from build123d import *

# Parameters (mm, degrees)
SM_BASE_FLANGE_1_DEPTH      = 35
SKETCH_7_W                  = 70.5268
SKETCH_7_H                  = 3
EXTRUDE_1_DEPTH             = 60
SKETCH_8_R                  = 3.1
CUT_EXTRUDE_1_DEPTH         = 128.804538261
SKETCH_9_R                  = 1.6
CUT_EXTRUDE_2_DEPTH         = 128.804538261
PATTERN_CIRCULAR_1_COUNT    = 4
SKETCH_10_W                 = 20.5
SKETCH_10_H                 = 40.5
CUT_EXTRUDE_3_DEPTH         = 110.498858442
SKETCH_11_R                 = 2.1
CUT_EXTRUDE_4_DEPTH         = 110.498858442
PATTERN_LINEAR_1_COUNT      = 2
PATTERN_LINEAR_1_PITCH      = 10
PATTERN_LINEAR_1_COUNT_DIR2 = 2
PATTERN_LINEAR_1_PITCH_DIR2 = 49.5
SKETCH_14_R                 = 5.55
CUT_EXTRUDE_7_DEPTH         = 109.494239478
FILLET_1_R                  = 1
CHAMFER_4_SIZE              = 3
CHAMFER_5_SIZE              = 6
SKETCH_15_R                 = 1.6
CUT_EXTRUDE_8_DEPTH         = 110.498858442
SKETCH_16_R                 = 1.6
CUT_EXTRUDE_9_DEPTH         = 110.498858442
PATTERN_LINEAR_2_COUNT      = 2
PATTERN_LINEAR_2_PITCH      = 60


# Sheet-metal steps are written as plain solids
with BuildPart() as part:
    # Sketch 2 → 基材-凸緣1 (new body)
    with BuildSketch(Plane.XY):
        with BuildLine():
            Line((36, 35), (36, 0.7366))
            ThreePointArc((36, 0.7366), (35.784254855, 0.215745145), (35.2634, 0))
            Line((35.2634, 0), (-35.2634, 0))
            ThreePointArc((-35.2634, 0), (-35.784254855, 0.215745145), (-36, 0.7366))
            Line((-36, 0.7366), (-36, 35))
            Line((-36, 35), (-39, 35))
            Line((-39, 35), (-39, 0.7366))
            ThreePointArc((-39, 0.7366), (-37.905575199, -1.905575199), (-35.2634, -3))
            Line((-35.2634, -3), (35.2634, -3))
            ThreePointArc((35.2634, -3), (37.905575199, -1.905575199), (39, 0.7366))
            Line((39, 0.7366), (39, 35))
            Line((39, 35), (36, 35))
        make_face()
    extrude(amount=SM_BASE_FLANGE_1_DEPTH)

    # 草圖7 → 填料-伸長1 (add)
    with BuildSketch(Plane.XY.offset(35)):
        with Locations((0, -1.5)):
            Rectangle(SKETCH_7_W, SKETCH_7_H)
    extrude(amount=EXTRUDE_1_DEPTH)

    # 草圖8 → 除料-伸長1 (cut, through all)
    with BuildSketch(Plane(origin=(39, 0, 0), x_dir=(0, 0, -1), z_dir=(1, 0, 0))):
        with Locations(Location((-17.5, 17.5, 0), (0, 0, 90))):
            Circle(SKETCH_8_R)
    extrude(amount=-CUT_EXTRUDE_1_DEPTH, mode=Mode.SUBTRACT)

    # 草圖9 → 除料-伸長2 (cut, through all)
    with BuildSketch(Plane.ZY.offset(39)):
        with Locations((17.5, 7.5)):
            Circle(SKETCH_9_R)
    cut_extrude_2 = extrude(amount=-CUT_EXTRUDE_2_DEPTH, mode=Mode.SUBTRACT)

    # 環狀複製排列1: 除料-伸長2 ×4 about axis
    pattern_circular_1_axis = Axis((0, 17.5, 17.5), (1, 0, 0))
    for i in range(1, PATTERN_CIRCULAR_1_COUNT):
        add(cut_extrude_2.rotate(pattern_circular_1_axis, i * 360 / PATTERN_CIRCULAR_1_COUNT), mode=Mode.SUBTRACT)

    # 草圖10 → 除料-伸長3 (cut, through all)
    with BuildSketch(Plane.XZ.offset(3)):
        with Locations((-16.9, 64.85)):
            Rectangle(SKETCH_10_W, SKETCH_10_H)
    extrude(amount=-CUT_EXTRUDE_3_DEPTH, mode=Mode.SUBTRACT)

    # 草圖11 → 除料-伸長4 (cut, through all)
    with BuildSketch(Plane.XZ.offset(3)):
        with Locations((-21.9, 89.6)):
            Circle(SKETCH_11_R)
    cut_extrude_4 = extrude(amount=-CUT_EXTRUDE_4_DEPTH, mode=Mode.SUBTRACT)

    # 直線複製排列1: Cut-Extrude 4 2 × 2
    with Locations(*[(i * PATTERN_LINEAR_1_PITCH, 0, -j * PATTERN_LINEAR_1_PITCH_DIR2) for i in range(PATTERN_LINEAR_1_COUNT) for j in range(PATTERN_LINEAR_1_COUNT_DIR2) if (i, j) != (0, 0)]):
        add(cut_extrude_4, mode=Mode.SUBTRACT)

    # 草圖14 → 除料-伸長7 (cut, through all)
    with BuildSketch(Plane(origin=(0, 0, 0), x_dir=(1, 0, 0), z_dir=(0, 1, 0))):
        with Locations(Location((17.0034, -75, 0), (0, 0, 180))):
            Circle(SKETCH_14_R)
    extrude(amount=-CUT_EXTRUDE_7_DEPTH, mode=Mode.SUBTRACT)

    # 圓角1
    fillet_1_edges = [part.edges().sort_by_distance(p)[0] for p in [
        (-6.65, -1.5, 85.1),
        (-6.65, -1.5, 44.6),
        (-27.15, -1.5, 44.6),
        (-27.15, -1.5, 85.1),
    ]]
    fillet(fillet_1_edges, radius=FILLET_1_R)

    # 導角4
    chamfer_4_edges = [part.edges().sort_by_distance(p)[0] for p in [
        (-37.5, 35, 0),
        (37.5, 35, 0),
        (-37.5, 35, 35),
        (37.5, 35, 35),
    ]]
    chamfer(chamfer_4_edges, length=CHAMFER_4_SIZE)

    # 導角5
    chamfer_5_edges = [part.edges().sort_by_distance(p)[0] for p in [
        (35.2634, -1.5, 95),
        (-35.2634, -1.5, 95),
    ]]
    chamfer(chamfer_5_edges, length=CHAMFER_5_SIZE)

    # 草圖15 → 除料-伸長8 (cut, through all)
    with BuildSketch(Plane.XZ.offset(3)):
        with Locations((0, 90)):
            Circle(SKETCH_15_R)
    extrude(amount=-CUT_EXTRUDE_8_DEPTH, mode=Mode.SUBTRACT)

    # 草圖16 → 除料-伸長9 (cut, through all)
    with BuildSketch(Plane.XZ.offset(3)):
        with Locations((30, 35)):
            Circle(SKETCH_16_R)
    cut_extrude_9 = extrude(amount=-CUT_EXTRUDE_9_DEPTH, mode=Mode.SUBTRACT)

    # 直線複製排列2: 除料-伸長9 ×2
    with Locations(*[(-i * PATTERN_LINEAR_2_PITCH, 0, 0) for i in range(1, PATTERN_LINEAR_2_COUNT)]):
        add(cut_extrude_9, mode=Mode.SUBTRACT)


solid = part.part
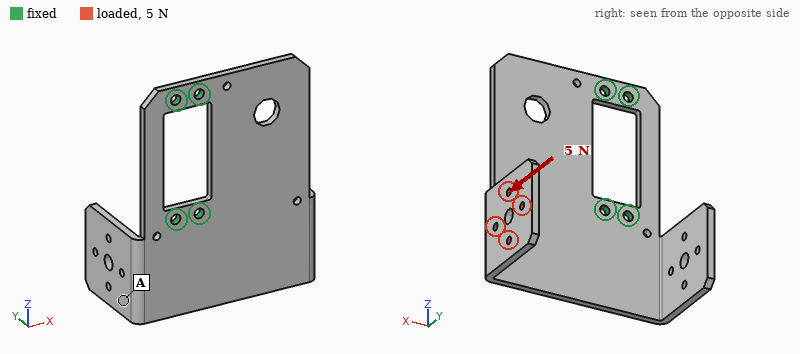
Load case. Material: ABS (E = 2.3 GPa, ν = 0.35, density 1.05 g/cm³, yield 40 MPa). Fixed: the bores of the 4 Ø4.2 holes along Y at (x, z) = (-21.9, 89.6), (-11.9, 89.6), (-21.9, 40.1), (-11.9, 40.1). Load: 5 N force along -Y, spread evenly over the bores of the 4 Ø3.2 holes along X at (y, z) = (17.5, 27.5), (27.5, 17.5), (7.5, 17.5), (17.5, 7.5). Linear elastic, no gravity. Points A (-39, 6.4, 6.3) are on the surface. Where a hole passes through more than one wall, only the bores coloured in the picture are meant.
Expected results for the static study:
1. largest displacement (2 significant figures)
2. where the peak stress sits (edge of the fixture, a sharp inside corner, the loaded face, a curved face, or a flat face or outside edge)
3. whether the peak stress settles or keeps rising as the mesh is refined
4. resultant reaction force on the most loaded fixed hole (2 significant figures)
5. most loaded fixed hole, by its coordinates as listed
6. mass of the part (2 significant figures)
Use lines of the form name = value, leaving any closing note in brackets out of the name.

largest displacement = 1.5 mm
where the peak stress sits = edge of the fixture
whether the peak stress settles or keeps rising as the mesh is refined = keeps rising
resultant reaction force on the most loaded fixed hole = 14 N
most loaded fixed hole, by its coordinates as listed = (-11.9, 40.1)
mass of the part = 26 g
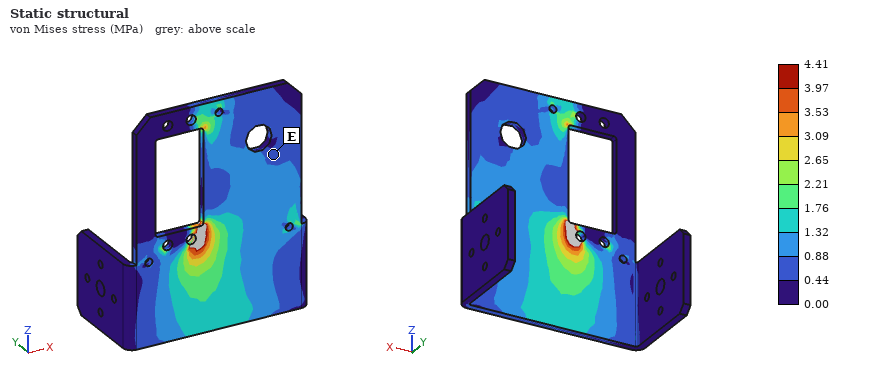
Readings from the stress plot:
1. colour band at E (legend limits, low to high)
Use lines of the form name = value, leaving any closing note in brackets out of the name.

colour band at E = 0.44 to 0.88 MPa
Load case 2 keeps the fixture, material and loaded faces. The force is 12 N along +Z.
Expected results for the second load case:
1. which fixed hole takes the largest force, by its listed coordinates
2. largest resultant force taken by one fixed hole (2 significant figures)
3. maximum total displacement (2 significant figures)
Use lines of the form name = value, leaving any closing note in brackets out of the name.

which fixed hole takes the largest force, by its listed coordinates = (-11.9, 40.1)
largest resultant force taken by one fixed hole = 14 N
maximum total displacement = 1.4 mm
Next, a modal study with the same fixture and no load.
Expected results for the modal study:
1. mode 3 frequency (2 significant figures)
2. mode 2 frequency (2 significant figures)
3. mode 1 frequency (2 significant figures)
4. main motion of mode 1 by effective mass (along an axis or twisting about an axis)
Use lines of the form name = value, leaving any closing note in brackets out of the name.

mode 3 frequency = 270 Hz
mode 2 frequency = 220 Hz
mode 1 frequency = 130 Hz
main motion of mode 1 by effective mass = along Y
